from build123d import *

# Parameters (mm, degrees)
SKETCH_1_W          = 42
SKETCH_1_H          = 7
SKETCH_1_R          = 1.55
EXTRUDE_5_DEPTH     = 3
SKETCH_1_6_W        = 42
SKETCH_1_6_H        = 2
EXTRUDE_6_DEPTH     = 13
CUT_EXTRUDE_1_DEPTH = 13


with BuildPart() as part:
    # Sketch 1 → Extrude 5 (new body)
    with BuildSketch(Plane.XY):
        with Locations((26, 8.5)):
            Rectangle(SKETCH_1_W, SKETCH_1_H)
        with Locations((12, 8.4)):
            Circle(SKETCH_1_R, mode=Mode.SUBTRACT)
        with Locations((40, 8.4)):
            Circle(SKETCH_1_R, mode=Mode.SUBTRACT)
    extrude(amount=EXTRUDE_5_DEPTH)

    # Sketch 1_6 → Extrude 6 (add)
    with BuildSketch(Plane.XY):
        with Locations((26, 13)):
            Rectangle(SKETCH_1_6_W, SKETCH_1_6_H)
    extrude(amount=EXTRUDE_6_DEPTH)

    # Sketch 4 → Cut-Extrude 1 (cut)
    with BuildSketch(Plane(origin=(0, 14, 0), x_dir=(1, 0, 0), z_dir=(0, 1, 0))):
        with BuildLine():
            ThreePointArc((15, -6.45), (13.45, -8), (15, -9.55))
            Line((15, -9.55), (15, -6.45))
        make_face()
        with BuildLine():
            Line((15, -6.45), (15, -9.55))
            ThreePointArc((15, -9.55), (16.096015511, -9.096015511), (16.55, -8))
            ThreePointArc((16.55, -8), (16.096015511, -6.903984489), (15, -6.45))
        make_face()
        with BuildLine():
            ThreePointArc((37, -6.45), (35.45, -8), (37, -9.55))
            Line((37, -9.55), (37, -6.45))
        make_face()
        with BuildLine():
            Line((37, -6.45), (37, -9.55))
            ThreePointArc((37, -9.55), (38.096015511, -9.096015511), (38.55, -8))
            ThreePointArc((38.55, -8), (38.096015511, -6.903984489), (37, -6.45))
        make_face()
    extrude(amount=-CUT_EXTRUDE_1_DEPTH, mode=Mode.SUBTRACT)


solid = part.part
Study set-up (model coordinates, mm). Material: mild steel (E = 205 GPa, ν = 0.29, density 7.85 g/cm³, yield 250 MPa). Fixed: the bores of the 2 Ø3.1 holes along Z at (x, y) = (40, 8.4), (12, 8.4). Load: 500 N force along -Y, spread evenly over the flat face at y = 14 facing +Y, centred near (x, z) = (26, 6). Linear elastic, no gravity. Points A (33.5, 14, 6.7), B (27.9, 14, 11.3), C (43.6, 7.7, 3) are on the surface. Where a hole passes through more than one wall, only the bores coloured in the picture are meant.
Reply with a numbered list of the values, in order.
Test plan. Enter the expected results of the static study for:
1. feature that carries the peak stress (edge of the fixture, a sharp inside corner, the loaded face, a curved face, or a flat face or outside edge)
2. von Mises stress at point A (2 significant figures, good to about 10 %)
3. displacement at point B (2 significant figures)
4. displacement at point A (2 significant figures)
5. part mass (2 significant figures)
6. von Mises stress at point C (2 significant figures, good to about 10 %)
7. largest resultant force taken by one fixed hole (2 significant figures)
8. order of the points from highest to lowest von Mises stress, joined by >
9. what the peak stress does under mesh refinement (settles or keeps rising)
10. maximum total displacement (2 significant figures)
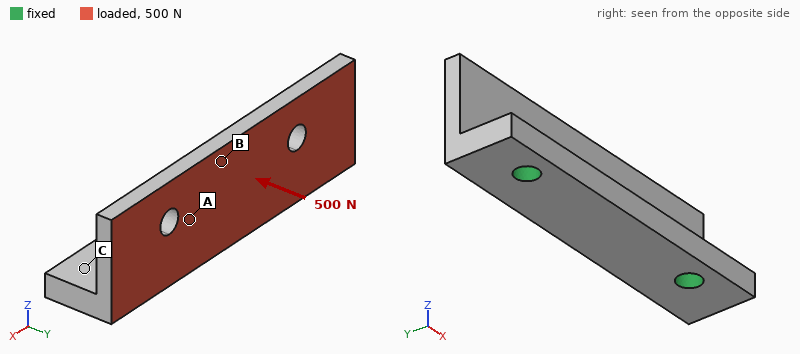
1. edge of the fixture
2. 30 MPa
3. 19 µm
4. 9.1 µm
5. 15 g
6. 19 MPa
7. 250 N
8. A > C > B
9. keeps rising
10. 23 µm
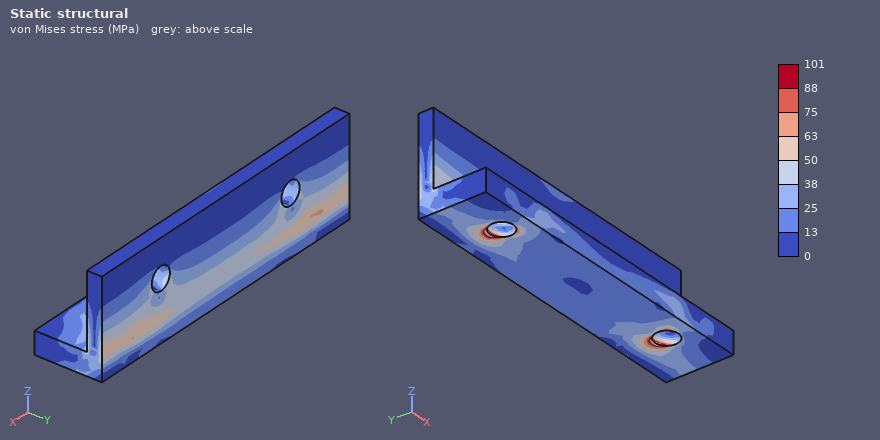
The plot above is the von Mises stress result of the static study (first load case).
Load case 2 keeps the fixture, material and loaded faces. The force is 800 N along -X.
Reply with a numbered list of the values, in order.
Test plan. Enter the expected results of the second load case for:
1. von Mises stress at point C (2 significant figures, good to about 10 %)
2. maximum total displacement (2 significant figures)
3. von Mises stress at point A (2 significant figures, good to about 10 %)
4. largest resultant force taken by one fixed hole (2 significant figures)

1. 6.4 MPa
2. 3.1 µm
3. 11 MPa
4. 440 N
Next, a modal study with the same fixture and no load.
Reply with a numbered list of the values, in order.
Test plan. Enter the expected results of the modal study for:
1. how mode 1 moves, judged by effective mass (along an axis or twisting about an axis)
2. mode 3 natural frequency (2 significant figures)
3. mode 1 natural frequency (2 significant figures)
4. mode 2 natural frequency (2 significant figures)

1. along Y
2. 18 kHz
3. 10 kHz
4. 13 kHz
